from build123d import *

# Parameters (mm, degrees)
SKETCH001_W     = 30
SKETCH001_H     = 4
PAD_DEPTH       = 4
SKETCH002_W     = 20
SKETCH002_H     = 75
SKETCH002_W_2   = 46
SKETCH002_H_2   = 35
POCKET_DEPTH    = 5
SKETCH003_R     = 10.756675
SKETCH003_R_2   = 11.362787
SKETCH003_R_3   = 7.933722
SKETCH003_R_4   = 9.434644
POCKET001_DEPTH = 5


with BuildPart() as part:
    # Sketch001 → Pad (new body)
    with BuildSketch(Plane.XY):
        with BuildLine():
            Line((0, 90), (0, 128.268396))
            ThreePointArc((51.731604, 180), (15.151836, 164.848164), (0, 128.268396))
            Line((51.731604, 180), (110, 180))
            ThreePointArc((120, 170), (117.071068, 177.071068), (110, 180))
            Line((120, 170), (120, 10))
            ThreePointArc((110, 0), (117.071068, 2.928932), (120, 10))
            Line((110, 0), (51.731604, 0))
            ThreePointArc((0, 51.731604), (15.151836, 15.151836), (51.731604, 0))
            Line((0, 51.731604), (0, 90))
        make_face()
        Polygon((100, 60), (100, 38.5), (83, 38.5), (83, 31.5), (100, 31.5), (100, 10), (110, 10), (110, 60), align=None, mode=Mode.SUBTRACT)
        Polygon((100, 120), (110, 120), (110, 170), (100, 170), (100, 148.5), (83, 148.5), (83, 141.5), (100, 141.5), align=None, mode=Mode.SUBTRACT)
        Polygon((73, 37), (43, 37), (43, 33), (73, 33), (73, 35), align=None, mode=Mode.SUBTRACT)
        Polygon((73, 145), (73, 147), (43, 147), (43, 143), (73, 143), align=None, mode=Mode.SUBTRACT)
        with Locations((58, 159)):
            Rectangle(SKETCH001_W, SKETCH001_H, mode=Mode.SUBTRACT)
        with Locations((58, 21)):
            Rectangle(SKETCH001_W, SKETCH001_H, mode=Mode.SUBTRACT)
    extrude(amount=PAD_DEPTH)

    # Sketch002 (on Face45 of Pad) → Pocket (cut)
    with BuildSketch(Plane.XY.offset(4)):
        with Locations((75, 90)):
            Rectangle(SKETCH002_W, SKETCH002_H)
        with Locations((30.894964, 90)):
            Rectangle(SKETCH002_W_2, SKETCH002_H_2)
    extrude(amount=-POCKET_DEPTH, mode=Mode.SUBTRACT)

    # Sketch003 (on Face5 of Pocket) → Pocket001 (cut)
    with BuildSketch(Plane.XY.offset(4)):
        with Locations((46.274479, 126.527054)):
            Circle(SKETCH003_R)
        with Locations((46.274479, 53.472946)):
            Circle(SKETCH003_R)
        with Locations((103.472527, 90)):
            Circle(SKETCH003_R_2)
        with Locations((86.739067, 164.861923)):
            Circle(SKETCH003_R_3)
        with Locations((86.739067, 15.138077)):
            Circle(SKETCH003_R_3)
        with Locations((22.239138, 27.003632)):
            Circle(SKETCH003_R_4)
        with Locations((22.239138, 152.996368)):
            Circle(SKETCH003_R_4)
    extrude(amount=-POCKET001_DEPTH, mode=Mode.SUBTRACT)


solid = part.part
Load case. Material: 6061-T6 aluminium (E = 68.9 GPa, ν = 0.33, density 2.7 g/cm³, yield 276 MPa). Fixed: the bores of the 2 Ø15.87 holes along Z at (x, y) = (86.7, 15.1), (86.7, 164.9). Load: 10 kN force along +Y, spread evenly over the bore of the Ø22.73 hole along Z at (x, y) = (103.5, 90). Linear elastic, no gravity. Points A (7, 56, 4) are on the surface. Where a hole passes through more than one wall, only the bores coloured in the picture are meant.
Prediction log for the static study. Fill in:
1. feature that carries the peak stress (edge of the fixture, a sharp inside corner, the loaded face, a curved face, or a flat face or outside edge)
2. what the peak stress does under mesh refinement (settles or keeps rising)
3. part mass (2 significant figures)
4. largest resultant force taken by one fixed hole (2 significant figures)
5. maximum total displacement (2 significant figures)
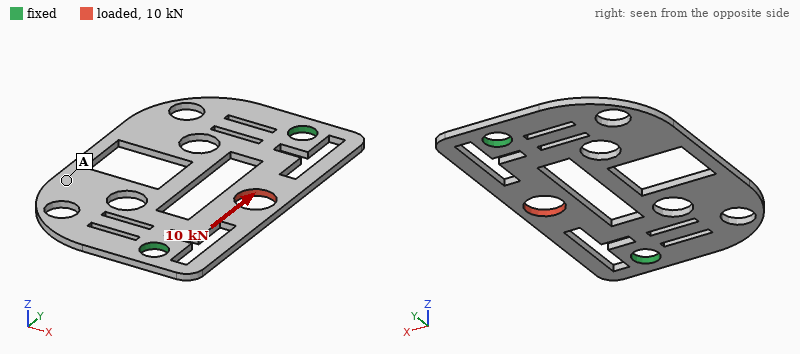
a sharp inside corner
keeps rising
150 g
5.2 kN
0.14 mm
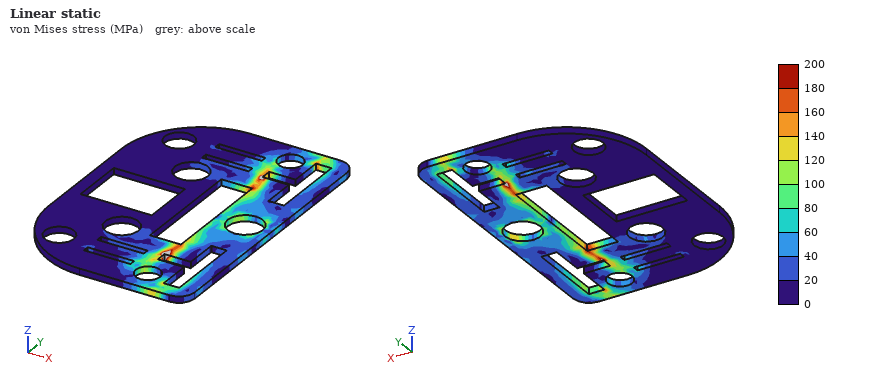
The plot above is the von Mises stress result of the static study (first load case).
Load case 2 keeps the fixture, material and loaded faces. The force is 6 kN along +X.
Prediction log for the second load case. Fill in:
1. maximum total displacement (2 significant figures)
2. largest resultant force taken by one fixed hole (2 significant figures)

0.21 mm
3.1 kN
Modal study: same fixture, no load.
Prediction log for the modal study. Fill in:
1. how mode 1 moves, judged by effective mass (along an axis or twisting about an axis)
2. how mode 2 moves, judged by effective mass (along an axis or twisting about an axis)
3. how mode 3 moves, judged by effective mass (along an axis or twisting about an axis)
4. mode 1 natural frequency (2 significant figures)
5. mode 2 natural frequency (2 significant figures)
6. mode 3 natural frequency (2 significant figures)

along Z
along Z
twisting about X
370 Hz
740 Hz
790 Hz
